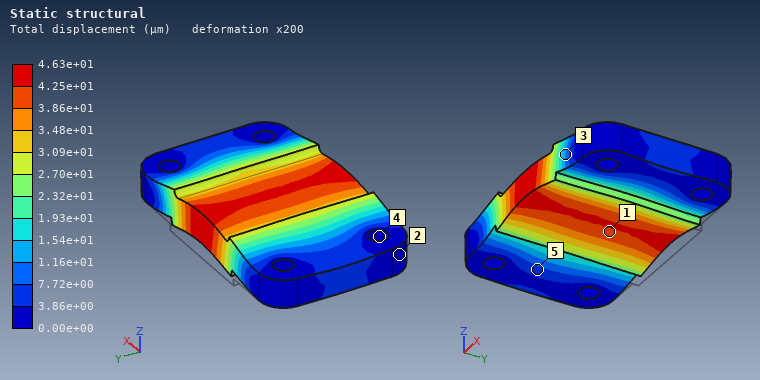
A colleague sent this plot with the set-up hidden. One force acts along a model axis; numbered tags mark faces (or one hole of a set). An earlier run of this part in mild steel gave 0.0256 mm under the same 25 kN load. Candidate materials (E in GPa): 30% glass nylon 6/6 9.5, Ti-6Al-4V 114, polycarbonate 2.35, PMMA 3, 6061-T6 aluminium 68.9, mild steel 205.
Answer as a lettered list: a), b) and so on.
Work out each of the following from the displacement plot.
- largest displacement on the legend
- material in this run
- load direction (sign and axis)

a) 4.63e+01 µm
b) Ti-6Al-4V
c) +Z
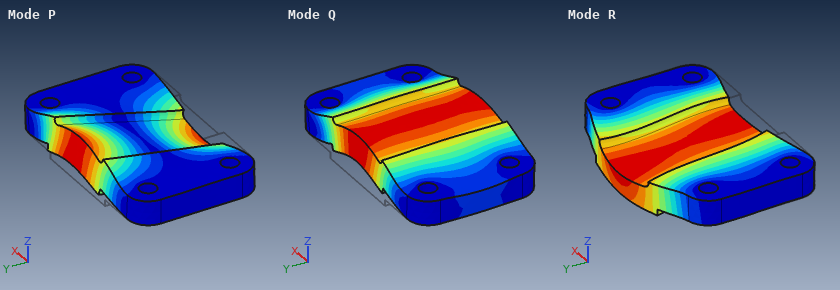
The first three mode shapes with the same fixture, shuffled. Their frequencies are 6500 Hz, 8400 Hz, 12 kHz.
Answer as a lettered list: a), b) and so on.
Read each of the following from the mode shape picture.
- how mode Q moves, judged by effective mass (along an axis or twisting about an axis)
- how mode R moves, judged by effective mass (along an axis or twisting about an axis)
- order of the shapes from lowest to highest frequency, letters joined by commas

a) along Z
b) along Y
c) Q, P, R
